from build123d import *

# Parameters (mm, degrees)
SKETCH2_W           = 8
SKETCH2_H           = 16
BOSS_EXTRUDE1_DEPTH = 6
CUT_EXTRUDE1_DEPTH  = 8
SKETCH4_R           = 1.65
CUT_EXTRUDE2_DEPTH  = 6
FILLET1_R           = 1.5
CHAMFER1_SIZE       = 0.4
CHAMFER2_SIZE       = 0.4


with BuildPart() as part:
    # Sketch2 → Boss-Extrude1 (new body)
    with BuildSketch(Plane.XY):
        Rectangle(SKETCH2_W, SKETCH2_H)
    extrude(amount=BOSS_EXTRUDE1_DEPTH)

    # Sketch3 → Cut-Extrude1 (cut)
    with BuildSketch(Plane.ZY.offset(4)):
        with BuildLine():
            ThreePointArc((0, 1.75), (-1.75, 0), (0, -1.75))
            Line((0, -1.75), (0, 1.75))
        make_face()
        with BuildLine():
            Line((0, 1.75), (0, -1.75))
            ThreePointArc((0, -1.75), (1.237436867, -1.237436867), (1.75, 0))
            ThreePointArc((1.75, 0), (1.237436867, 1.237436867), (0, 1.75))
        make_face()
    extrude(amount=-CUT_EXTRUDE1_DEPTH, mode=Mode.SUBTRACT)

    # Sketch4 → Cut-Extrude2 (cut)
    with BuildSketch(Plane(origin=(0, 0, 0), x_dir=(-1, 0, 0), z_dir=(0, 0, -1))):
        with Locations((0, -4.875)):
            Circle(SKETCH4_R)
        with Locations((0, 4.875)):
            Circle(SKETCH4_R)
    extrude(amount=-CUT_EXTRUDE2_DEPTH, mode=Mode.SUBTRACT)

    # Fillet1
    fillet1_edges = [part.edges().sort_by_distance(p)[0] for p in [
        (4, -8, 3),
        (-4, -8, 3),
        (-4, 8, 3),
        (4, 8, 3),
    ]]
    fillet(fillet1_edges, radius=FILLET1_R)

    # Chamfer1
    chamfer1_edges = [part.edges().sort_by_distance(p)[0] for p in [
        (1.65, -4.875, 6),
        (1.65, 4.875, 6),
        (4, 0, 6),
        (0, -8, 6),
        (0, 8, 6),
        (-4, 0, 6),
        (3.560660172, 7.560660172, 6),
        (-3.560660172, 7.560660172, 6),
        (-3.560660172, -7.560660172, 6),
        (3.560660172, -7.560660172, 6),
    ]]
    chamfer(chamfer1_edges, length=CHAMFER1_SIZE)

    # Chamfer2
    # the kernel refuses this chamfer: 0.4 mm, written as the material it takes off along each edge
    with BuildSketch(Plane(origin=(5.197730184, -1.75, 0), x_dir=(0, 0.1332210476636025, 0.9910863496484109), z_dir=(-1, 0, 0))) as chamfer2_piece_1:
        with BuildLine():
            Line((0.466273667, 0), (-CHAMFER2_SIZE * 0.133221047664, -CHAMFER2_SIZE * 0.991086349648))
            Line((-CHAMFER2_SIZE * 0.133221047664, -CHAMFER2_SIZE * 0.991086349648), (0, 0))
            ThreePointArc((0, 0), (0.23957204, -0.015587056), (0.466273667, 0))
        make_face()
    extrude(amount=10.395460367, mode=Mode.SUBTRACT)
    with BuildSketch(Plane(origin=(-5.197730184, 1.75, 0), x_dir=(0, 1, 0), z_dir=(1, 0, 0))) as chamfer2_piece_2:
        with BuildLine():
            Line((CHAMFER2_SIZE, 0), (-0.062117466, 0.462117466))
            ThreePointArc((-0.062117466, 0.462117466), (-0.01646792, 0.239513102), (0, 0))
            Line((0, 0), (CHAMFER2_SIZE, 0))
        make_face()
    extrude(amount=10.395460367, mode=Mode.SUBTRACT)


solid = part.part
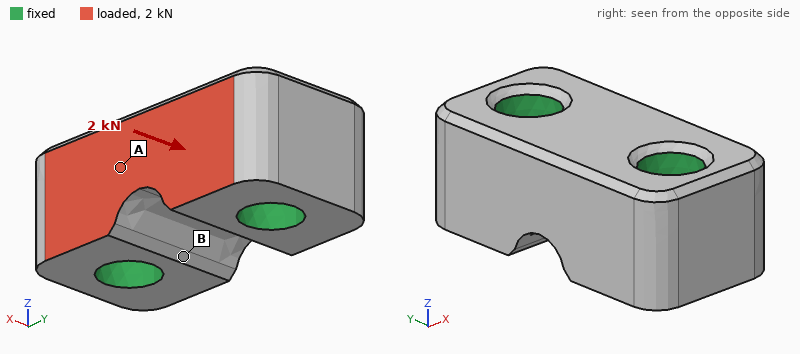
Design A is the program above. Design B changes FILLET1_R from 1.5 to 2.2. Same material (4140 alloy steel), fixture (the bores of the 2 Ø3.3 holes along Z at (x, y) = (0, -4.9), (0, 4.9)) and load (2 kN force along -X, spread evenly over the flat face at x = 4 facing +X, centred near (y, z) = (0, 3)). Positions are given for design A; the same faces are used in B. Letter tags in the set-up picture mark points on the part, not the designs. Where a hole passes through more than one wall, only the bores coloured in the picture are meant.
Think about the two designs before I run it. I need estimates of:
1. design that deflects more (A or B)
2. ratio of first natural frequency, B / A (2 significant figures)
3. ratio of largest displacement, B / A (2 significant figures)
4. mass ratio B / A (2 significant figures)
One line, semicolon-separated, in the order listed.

B; 1.0; 1.2; 0.98
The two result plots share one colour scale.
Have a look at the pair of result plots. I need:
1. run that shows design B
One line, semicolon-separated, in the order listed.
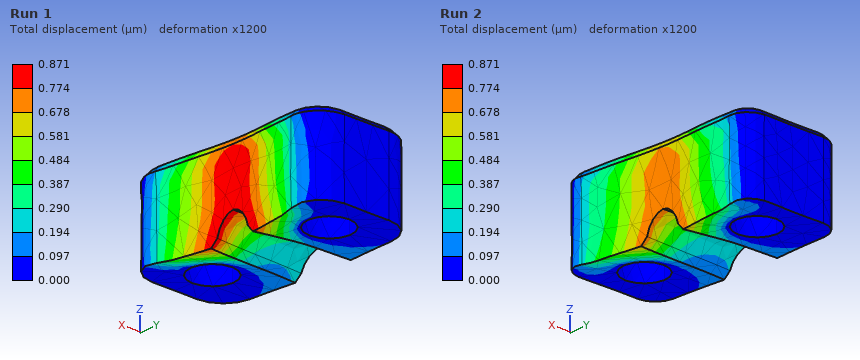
Run 1
